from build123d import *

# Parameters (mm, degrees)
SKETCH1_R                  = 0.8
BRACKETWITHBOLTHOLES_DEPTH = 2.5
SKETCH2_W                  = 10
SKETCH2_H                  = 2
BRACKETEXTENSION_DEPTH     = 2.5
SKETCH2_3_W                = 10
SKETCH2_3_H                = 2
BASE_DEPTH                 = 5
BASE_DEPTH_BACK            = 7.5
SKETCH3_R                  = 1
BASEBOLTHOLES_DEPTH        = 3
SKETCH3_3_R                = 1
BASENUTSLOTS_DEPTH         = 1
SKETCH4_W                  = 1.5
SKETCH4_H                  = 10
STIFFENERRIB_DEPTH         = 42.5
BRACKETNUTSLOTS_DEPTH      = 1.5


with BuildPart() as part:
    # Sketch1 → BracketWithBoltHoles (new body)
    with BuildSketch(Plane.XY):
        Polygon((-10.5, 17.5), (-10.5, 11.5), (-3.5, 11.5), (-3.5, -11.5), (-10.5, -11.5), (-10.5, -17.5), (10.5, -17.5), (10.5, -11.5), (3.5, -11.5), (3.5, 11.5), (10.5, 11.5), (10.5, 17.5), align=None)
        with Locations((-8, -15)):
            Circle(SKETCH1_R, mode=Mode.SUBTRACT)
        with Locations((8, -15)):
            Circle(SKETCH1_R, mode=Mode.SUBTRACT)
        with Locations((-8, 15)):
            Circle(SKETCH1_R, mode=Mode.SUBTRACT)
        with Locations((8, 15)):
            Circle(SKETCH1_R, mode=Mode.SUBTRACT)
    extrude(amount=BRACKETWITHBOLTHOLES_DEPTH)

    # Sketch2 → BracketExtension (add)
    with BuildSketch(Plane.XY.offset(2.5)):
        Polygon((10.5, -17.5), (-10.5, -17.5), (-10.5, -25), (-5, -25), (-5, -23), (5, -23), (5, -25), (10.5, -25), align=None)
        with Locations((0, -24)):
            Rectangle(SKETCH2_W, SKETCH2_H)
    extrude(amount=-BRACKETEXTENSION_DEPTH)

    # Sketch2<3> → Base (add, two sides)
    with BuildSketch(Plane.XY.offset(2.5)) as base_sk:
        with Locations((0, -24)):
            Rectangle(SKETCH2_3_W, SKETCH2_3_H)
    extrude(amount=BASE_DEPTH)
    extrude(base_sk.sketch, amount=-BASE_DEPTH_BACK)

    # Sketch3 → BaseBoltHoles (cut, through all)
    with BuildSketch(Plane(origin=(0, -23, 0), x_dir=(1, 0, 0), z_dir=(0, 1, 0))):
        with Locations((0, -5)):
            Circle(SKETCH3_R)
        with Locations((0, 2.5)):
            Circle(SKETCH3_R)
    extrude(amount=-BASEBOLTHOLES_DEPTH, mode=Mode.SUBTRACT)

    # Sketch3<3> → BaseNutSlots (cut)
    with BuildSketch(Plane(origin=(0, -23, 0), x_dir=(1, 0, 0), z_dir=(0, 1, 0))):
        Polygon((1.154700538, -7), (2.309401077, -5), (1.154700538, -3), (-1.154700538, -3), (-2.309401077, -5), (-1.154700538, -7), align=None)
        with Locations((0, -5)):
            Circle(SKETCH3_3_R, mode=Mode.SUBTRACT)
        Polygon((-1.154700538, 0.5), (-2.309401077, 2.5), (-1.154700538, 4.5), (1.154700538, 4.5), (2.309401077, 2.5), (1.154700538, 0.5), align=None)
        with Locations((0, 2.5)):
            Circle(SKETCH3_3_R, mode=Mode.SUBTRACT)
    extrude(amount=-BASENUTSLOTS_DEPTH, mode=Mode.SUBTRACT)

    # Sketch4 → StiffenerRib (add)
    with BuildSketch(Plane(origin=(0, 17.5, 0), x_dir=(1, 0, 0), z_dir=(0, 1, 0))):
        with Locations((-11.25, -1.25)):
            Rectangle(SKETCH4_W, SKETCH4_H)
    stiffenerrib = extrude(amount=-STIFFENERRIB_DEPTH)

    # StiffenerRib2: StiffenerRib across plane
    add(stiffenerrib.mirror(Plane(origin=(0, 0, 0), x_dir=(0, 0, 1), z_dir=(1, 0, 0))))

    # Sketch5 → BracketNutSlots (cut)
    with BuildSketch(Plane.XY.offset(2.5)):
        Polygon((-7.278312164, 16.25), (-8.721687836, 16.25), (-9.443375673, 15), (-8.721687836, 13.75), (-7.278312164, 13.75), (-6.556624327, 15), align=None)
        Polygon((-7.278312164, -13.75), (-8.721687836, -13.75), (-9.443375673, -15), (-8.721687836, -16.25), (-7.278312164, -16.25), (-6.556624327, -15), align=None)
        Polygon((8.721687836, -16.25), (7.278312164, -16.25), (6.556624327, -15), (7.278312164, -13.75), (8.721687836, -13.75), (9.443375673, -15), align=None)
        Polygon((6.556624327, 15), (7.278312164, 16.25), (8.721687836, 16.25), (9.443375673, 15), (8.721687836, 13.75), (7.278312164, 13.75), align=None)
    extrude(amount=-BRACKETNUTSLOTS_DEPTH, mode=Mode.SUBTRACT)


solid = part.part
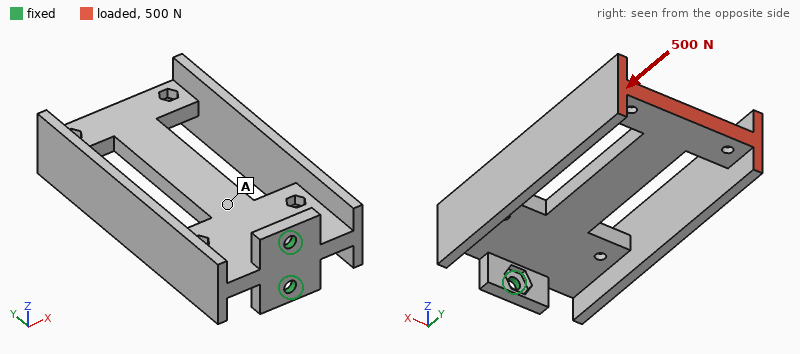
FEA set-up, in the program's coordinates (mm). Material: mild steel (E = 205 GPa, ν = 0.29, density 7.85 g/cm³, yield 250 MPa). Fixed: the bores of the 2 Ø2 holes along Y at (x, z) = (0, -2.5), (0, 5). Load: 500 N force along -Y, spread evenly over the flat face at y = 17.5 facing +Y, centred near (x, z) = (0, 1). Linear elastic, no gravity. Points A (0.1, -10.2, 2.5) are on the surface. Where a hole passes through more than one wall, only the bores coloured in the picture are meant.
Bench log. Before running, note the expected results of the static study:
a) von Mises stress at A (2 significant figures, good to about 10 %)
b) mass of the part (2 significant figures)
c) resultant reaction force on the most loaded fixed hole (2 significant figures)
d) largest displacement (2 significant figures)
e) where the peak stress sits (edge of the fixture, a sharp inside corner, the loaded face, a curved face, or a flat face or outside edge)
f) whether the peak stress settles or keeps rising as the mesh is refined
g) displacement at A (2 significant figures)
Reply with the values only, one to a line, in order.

14 MPa
22 g
280 N
5.2 µm
edge of the fixture
keeps rising
3.2 µm
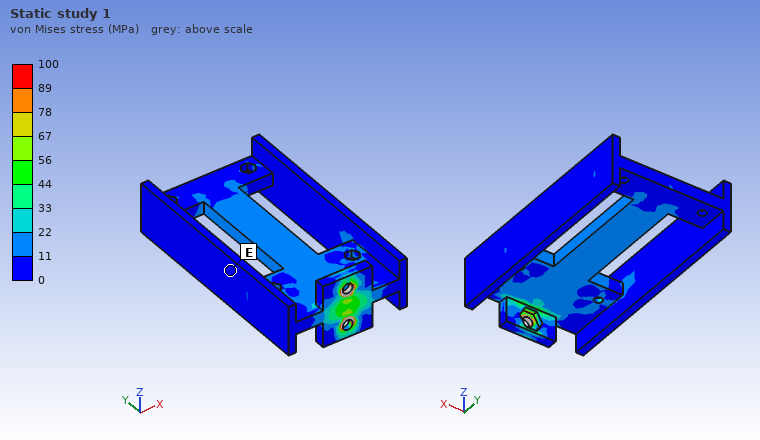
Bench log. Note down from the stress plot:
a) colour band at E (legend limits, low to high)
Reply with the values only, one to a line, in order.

0 to 11 MPa
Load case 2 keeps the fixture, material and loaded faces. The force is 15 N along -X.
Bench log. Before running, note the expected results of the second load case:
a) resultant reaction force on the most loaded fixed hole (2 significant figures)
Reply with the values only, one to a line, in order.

7.5 N
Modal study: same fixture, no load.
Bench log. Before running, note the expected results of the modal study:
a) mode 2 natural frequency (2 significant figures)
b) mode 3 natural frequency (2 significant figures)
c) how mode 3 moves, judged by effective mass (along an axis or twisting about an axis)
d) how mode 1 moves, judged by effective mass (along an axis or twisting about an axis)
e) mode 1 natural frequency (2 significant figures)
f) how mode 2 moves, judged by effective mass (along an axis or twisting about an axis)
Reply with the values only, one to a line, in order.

1200 Hz
2600 Hz
twisting about Y
along X
1000 Hz
along Z
